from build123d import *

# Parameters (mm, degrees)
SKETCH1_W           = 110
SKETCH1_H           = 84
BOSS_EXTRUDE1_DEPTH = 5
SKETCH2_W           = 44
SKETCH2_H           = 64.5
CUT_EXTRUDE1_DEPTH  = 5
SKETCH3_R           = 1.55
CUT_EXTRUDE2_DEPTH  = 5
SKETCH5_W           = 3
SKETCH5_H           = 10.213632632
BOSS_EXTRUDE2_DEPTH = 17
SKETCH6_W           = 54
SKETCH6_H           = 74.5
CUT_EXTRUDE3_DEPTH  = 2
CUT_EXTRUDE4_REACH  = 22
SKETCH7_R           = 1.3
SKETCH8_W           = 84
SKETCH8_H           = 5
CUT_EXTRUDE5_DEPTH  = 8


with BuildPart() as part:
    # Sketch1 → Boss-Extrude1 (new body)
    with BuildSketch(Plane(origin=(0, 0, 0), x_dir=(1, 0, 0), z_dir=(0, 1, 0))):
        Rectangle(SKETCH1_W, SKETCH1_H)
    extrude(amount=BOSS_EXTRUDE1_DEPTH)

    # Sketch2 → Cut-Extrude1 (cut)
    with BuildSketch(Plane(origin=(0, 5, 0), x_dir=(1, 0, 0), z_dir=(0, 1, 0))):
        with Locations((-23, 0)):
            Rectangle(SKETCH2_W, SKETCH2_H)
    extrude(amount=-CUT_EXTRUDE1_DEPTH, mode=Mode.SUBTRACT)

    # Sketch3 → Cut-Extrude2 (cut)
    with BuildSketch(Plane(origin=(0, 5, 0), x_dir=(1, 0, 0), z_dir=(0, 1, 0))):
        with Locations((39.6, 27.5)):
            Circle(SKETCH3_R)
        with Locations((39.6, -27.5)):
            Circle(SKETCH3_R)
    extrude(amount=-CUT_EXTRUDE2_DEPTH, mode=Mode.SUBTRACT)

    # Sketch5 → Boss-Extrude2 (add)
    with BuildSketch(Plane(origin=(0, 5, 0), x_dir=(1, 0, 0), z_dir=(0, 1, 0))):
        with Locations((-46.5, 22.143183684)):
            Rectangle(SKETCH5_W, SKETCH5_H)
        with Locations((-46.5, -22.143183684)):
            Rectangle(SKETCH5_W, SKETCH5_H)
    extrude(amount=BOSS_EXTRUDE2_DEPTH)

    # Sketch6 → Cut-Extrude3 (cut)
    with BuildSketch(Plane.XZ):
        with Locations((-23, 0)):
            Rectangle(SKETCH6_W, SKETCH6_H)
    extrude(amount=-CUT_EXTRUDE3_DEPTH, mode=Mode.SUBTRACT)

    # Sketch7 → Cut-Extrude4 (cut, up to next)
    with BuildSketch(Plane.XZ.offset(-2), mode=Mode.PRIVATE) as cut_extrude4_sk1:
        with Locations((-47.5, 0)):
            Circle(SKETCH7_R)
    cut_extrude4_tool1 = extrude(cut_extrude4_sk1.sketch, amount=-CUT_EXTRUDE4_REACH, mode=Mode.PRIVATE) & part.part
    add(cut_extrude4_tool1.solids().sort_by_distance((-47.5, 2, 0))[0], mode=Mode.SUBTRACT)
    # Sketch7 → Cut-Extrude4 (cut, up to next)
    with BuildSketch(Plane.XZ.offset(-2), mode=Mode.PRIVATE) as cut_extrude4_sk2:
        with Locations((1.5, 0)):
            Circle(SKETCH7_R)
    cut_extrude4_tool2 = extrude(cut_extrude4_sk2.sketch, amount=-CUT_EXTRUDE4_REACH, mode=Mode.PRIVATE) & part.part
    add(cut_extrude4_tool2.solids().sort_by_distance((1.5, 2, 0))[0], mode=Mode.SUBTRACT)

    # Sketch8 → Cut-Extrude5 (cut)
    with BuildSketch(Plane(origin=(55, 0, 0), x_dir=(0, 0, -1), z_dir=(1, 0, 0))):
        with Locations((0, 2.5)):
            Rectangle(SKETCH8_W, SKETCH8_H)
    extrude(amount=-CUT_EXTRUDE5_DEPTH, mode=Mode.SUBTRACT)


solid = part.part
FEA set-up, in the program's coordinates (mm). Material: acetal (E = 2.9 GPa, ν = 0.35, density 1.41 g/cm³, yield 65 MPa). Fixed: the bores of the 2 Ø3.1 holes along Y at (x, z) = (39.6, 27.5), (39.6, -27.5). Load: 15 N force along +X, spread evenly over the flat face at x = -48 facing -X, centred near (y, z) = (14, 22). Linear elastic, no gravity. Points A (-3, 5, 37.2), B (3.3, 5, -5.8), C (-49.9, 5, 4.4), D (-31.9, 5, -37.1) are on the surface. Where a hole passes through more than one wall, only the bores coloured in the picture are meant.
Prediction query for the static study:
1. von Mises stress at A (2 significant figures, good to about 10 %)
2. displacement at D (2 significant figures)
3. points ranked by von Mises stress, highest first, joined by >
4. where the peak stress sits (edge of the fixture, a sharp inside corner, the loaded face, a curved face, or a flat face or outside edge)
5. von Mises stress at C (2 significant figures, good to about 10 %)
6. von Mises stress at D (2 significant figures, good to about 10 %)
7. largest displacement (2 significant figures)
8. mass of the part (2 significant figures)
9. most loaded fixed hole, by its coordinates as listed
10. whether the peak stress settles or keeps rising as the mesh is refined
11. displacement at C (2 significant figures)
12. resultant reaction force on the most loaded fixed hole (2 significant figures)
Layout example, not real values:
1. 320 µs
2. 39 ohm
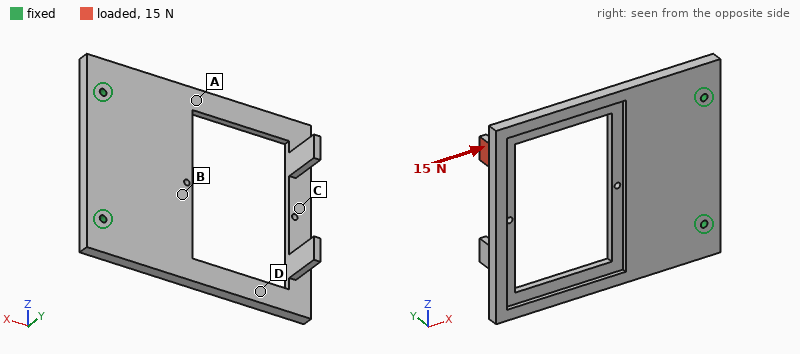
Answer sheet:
1. 3.1 MPa
2. 0.41 mm
3. A > C > D > B
4. a sharp inside corner
5. 2.4 MPa
6. 1.8 MPa
7. 1.3 mm
8. 38 g
9. (39.6, 27.5)
10. keeps rising
11. 0.86 mm
12. 13 N
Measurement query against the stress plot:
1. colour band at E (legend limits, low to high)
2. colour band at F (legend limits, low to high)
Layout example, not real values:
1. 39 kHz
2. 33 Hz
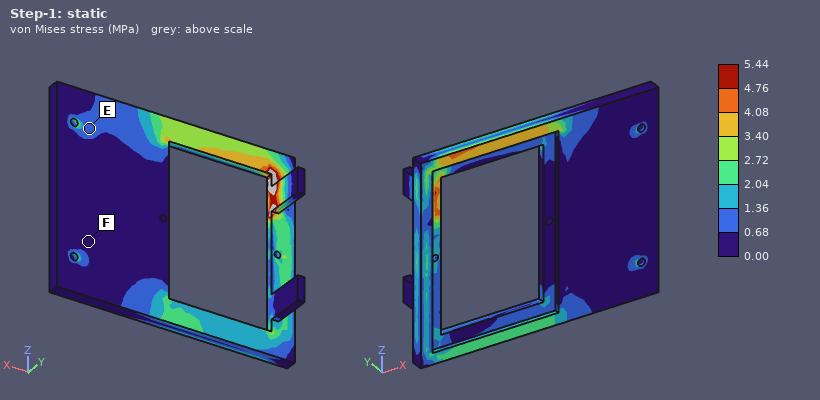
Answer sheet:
1. 0.68 to 1.36 MPa
2. 0.00 to 0.68 MPa
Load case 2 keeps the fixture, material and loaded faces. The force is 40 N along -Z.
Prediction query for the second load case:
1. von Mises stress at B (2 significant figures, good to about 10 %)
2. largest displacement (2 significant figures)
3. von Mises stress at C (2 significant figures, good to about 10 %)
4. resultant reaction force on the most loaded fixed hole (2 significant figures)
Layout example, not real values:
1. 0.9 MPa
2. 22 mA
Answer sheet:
1. 1.2 MPa
2. 1.5 mm
3. 7.3 MPa
4. 66 N
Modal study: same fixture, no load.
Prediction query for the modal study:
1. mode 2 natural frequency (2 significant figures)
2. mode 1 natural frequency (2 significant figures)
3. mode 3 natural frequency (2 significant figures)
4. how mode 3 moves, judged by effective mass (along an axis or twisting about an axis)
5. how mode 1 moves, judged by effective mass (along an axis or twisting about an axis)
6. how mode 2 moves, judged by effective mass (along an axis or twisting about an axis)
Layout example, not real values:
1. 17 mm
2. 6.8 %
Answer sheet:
1. 230 Hz
2. 110 Hz
3. 490 Hz
4. along Z
5. along Y
6. twisting about X
